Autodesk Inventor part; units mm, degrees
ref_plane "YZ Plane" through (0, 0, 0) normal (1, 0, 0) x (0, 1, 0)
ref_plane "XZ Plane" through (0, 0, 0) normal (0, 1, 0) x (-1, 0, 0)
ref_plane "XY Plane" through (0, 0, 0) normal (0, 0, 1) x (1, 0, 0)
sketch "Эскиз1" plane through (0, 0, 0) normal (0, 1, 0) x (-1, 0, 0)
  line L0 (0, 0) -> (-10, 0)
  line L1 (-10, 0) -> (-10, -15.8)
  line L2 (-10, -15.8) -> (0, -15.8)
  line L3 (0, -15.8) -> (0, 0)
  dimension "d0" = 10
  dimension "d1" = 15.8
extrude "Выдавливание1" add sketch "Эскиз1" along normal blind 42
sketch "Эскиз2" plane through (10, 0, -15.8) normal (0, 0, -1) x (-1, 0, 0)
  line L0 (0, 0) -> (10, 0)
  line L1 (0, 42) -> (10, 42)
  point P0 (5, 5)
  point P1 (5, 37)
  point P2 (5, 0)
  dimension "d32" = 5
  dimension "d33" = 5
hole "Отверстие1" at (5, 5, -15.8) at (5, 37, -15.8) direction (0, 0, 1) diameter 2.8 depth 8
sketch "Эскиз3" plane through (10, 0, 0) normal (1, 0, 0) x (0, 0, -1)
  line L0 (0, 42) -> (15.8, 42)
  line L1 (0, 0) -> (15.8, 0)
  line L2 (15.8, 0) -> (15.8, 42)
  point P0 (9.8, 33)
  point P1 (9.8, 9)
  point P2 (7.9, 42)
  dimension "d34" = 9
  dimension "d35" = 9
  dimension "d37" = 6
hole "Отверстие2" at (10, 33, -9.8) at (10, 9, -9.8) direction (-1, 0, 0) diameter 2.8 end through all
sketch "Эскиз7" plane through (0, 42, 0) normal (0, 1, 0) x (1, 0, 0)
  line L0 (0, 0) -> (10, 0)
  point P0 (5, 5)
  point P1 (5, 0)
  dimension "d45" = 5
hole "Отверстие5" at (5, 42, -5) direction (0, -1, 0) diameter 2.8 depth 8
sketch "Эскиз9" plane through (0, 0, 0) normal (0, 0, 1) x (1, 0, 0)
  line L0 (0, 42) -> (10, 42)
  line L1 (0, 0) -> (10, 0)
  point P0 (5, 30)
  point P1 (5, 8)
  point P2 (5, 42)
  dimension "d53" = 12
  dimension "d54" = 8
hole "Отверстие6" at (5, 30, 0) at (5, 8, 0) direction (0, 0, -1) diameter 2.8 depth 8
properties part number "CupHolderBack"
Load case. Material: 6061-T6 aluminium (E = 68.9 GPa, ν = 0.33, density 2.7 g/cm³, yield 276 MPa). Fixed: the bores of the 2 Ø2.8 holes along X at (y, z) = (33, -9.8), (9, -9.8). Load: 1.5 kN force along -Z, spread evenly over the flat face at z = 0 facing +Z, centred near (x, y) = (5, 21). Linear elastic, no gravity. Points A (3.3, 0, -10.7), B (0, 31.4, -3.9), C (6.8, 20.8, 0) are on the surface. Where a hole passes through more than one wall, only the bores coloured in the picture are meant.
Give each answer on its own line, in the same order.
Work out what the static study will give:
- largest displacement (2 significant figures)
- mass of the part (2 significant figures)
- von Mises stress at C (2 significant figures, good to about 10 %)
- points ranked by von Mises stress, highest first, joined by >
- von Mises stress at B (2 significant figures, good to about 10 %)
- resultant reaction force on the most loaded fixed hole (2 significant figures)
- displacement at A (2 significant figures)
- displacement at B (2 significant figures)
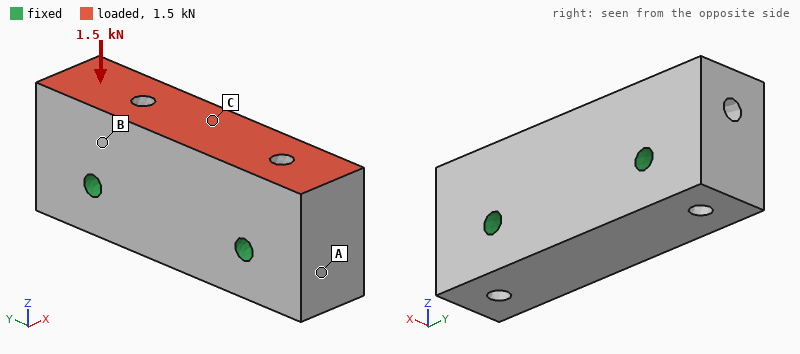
1.5 µm
17 g
3.3 MPa
B > C > A
5.6 MPa
760 N
0.85 µm
0.57 µm
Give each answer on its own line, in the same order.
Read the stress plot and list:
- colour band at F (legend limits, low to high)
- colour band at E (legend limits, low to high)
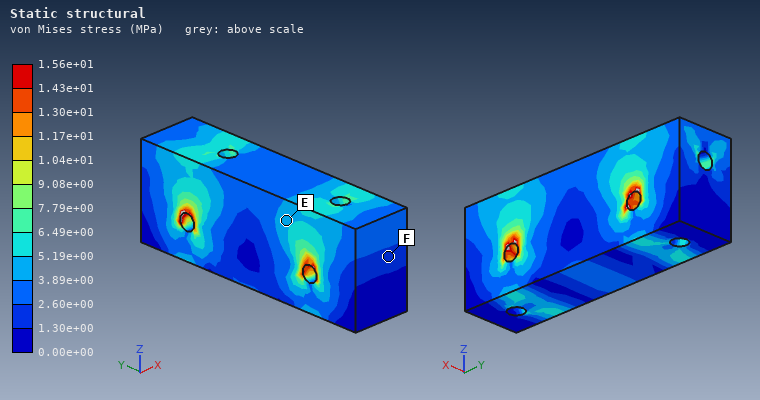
1.30e+00 to 2.60e+00 MPa
3.89e+00 to 5.19e+00 MPa
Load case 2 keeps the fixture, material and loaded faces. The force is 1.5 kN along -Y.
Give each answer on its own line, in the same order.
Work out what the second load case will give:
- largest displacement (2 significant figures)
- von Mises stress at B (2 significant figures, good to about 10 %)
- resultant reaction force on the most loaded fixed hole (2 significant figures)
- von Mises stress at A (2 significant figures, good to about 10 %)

4.9 µm
9.3 MPa
930 N
3.4 MPa
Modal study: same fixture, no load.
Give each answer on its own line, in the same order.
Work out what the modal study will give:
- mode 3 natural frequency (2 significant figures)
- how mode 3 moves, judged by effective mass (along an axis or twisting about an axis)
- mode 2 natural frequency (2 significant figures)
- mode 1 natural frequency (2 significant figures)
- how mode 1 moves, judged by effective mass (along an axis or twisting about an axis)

42 kHz
twisting about Z
39 kHz
34 kHz
along X
